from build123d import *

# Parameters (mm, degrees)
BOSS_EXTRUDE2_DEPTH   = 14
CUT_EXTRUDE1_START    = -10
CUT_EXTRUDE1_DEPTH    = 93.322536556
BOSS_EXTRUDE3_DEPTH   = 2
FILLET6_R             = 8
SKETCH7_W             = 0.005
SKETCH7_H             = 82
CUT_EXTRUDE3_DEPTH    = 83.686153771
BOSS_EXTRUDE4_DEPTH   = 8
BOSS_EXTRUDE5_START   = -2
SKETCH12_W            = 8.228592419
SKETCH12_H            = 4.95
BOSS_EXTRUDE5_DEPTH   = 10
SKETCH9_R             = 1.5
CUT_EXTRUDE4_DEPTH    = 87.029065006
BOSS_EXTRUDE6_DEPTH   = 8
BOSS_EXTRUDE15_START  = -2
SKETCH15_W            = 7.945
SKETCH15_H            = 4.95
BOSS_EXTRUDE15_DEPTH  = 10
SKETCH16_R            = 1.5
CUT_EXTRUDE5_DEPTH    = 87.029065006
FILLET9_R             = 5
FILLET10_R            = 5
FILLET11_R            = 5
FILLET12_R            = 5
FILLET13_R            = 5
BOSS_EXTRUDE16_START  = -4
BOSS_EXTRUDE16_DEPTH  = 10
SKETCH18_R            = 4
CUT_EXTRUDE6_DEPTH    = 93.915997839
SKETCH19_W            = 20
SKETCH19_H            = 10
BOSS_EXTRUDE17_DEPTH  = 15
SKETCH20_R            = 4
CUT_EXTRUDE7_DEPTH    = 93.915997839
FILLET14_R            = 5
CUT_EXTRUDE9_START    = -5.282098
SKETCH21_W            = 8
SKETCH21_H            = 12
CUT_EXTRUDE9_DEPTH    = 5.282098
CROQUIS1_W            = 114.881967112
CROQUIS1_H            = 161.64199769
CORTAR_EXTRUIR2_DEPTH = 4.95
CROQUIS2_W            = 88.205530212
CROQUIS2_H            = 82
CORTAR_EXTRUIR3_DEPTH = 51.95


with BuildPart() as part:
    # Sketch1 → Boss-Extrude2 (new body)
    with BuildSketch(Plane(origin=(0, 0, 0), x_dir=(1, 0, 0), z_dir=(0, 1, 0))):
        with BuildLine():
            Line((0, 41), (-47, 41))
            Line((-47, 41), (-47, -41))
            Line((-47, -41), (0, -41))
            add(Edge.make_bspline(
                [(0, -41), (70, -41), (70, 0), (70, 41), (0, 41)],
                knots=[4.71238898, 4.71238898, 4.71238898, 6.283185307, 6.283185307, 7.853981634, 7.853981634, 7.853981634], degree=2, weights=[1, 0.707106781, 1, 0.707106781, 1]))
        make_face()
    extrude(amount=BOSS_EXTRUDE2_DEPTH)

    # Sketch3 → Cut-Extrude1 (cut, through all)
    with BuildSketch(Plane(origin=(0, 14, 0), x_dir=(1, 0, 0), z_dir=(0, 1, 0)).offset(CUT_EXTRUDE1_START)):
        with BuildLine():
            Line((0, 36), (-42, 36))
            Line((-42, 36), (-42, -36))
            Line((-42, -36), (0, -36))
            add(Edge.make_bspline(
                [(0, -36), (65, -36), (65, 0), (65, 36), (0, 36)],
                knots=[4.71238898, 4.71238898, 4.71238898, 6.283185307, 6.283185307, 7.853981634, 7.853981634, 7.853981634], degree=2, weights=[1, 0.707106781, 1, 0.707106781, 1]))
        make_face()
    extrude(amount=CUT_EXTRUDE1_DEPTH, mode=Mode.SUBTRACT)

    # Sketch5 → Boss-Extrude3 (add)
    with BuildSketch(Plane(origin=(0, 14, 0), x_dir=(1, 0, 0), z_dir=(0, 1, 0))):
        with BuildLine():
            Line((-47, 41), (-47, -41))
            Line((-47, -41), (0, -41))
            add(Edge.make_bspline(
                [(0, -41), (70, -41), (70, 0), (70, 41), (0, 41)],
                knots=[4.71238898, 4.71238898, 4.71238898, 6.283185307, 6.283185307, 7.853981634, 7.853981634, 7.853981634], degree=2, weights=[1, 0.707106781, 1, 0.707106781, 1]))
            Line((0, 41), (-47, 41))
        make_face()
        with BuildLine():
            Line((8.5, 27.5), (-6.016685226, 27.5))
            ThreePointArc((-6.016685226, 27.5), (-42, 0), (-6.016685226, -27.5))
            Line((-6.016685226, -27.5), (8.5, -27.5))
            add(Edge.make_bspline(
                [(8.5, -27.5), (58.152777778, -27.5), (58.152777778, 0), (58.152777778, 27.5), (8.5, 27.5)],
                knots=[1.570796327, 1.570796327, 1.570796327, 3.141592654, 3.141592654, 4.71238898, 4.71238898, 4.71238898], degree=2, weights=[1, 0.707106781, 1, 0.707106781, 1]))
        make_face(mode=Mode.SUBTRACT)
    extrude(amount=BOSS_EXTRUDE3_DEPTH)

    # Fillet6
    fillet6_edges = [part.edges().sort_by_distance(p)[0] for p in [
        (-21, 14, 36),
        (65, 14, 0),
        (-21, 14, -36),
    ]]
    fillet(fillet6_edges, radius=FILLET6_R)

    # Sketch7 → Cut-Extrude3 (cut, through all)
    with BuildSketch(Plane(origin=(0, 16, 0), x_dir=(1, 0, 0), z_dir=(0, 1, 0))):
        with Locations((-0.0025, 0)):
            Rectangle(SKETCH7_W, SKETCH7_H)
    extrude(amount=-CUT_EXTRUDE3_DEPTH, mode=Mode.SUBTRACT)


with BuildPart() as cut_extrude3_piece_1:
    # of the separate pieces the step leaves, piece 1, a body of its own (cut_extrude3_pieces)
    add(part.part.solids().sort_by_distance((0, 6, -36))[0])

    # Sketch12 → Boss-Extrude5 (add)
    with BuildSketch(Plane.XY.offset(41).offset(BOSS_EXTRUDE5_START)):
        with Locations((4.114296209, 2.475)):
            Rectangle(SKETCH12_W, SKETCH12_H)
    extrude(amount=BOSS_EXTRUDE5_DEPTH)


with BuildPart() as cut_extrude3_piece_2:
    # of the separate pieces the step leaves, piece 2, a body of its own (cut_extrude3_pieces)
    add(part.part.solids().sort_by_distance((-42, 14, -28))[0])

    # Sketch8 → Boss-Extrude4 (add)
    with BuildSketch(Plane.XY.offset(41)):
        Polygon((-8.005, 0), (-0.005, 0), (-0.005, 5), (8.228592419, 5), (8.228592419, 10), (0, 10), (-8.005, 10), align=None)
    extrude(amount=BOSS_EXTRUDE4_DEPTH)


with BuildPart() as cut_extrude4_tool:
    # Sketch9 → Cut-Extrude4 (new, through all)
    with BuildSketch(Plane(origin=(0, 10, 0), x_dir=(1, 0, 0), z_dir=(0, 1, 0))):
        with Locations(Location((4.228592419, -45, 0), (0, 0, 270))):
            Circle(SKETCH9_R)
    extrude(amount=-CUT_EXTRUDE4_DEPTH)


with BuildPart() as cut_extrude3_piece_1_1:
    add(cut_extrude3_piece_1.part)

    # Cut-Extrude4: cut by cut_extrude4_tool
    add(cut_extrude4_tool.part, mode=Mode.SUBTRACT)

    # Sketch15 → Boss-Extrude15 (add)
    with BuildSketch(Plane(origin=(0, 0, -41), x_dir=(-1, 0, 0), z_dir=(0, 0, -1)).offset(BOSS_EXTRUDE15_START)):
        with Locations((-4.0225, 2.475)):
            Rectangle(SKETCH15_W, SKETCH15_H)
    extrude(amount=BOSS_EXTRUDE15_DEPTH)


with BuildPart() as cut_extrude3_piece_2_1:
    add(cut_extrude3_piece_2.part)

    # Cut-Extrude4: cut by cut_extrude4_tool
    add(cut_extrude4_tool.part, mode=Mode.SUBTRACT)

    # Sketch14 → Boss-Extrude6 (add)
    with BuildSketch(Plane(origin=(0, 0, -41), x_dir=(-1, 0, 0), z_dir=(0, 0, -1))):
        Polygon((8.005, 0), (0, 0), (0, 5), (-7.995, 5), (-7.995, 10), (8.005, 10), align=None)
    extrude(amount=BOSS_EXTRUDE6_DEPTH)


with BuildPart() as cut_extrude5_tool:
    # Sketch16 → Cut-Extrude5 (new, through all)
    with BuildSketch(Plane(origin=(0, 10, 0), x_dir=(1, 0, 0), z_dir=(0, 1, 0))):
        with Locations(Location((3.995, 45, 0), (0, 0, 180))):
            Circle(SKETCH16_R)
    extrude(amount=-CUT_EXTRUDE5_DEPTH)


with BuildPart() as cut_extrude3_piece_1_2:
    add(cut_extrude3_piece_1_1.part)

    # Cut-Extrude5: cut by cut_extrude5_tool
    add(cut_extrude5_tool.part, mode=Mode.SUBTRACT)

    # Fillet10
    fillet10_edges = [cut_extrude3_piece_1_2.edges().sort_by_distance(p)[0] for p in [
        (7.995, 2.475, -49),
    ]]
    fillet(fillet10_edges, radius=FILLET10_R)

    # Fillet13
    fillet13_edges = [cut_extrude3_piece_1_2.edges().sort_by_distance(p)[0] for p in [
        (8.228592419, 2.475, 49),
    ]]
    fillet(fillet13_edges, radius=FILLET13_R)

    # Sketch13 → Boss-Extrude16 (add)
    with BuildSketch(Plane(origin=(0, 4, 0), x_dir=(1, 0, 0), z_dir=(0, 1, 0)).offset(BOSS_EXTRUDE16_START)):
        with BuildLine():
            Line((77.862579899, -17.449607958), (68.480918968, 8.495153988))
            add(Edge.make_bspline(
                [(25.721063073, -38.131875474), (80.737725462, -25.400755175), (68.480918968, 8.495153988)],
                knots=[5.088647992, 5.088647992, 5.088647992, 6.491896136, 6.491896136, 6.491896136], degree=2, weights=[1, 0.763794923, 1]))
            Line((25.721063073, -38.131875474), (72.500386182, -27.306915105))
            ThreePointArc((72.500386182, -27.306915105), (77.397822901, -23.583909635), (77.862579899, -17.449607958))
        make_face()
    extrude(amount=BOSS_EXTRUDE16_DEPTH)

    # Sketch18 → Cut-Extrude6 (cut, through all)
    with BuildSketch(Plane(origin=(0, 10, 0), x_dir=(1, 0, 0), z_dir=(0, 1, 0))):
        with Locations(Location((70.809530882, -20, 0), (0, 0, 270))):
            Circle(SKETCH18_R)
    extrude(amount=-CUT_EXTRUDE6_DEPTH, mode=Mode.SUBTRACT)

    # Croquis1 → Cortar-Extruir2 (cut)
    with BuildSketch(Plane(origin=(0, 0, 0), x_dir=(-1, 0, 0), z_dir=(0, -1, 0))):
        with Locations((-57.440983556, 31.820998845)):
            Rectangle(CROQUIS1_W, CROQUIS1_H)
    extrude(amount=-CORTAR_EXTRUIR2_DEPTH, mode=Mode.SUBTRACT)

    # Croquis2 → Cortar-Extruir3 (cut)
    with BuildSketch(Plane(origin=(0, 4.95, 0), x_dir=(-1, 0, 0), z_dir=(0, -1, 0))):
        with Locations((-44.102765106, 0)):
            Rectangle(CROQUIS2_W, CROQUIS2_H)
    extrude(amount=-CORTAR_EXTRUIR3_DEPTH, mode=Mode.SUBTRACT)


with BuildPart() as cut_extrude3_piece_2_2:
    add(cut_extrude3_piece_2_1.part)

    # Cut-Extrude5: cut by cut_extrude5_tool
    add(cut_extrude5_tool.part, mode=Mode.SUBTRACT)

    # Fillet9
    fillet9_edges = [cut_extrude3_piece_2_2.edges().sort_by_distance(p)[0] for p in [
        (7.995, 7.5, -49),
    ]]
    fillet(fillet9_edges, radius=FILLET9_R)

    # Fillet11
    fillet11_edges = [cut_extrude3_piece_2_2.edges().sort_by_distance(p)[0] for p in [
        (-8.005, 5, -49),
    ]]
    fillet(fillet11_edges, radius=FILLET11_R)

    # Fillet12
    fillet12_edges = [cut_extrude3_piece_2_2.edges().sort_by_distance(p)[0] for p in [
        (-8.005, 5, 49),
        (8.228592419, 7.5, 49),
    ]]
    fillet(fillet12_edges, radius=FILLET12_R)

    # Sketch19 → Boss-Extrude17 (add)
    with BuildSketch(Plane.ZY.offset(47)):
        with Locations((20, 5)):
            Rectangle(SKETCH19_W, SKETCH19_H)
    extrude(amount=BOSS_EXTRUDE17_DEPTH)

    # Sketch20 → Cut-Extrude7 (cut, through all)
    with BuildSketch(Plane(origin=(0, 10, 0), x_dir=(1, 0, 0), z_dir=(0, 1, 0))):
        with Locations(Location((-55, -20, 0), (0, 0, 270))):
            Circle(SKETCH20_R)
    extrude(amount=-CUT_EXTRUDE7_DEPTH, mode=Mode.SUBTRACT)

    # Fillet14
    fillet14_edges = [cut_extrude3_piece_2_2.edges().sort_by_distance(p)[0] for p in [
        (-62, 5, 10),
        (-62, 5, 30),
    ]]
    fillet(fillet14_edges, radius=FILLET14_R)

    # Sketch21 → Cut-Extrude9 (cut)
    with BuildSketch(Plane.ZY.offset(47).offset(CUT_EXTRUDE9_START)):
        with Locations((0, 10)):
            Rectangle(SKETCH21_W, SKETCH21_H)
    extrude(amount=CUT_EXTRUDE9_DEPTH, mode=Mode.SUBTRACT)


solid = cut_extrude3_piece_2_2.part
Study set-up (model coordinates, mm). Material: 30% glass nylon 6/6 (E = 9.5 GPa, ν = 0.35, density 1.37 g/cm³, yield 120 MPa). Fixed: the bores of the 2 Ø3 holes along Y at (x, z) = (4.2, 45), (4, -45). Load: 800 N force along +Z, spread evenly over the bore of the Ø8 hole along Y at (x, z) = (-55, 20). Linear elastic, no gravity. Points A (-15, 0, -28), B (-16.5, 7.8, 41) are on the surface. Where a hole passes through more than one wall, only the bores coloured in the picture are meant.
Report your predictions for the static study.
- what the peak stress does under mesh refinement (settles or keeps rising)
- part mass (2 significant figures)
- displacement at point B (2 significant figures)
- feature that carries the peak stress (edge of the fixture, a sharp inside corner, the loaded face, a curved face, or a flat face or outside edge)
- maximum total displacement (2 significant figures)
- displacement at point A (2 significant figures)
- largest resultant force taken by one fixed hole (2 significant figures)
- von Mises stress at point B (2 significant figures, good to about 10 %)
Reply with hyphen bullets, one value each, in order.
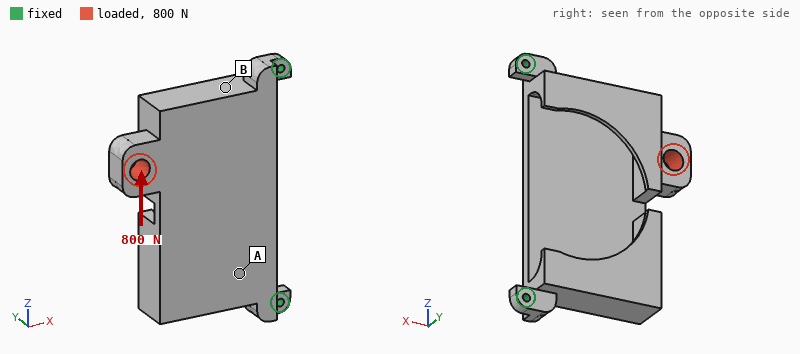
- keeps rising
- 44 g
- 0.14 mm
- edge of the fixture
- 0.45 mm
- 0.14 mm
- 640 N
- 9.5 MPa
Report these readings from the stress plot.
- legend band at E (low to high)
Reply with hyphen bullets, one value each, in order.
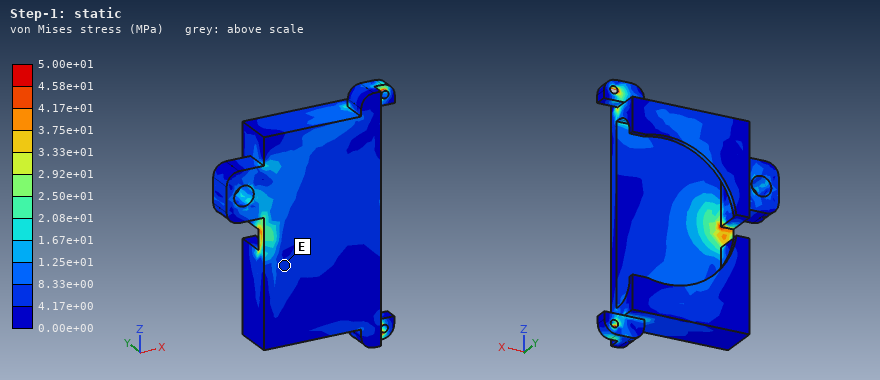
- 4.17e+00 to 8.33e+00 MPa
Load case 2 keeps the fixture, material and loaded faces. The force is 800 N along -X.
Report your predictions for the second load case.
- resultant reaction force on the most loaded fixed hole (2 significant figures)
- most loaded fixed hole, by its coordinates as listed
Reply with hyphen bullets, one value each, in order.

- 600 N
- (4.2, 45)
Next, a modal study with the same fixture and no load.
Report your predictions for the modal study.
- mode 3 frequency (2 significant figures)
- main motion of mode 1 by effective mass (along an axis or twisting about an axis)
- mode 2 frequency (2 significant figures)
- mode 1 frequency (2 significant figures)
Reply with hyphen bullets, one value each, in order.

- 1500 Hz
- along Y
- 970 Hz
- 340 Hz
